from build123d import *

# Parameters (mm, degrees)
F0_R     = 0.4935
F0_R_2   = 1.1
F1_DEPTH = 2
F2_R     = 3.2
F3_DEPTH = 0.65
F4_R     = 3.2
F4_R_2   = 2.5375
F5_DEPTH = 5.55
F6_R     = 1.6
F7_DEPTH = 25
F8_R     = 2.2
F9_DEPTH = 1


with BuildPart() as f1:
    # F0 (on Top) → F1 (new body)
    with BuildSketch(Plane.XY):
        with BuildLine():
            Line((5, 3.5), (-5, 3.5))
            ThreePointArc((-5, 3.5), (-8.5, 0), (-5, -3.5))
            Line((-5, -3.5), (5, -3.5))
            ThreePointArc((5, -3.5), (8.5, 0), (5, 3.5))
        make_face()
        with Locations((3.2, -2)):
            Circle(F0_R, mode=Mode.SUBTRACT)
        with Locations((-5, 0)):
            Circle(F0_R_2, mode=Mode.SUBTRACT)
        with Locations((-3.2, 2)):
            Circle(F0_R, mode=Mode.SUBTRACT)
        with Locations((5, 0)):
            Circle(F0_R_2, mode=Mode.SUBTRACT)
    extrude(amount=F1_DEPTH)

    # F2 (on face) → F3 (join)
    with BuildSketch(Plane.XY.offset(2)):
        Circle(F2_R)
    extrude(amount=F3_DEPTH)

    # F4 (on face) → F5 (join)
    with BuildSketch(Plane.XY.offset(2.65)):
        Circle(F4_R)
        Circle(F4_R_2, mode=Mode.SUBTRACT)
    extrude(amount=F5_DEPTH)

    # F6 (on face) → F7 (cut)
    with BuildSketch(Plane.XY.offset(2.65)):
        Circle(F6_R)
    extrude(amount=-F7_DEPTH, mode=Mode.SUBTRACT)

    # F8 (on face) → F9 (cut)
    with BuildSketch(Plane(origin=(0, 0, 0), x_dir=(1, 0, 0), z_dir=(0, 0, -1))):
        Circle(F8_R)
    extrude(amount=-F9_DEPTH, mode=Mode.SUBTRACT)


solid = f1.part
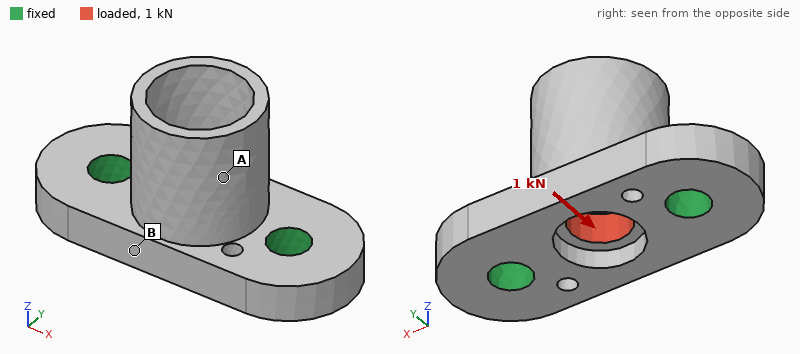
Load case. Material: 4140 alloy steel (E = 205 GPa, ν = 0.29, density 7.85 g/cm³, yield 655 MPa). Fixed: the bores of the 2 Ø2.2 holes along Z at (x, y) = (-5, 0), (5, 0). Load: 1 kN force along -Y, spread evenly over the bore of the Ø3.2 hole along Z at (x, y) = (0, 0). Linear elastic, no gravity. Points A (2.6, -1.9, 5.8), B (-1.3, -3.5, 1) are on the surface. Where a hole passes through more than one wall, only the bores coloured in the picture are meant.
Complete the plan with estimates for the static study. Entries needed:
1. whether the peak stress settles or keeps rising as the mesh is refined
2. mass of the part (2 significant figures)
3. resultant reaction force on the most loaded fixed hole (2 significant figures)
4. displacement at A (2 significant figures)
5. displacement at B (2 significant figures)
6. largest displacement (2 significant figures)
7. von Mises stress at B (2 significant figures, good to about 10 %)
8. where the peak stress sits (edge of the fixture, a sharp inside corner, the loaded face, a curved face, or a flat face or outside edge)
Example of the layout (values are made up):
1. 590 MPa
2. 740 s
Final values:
1. keeps rising
2. 2.0 g
3. 500 N
4. 4.9 µm
5. 3.0 µm
6. 6.5 µm
7. 74 MPa
8. edge of the fixture
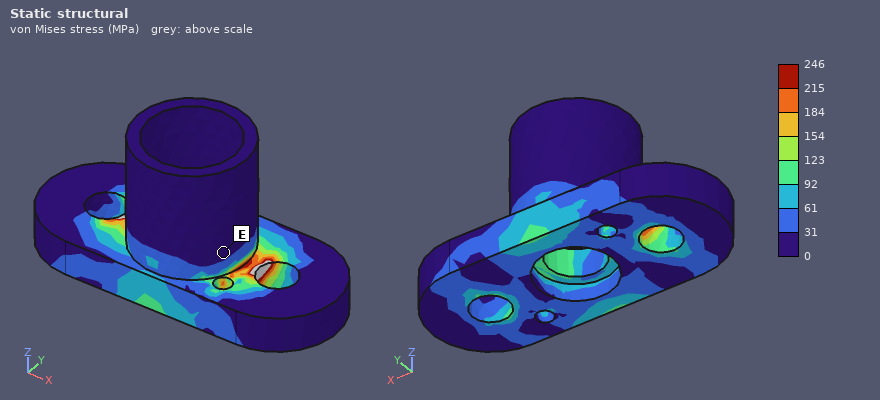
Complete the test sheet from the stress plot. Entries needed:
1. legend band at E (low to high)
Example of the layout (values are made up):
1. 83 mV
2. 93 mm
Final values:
1. 0 to 31 MPa
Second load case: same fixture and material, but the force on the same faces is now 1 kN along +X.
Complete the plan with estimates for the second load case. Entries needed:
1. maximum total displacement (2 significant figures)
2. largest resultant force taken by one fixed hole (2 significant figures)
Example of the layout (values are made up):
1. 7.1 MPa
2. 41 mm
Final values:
1. 1.4 µm
2. 510 N
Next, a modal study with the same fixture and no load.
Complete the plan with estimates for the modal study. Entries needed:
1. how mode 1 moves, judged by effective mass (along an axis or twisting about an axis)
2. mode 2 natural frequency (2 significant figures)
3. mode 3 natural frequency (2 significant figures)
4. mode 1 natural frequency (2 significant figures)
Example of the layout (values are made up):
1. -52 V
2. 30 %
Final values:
1. along Y
2. 61 kHz
3. 63 kHz
4. 36 kHz
